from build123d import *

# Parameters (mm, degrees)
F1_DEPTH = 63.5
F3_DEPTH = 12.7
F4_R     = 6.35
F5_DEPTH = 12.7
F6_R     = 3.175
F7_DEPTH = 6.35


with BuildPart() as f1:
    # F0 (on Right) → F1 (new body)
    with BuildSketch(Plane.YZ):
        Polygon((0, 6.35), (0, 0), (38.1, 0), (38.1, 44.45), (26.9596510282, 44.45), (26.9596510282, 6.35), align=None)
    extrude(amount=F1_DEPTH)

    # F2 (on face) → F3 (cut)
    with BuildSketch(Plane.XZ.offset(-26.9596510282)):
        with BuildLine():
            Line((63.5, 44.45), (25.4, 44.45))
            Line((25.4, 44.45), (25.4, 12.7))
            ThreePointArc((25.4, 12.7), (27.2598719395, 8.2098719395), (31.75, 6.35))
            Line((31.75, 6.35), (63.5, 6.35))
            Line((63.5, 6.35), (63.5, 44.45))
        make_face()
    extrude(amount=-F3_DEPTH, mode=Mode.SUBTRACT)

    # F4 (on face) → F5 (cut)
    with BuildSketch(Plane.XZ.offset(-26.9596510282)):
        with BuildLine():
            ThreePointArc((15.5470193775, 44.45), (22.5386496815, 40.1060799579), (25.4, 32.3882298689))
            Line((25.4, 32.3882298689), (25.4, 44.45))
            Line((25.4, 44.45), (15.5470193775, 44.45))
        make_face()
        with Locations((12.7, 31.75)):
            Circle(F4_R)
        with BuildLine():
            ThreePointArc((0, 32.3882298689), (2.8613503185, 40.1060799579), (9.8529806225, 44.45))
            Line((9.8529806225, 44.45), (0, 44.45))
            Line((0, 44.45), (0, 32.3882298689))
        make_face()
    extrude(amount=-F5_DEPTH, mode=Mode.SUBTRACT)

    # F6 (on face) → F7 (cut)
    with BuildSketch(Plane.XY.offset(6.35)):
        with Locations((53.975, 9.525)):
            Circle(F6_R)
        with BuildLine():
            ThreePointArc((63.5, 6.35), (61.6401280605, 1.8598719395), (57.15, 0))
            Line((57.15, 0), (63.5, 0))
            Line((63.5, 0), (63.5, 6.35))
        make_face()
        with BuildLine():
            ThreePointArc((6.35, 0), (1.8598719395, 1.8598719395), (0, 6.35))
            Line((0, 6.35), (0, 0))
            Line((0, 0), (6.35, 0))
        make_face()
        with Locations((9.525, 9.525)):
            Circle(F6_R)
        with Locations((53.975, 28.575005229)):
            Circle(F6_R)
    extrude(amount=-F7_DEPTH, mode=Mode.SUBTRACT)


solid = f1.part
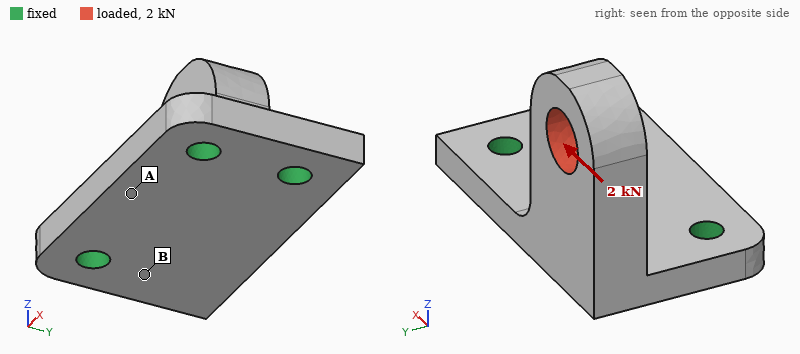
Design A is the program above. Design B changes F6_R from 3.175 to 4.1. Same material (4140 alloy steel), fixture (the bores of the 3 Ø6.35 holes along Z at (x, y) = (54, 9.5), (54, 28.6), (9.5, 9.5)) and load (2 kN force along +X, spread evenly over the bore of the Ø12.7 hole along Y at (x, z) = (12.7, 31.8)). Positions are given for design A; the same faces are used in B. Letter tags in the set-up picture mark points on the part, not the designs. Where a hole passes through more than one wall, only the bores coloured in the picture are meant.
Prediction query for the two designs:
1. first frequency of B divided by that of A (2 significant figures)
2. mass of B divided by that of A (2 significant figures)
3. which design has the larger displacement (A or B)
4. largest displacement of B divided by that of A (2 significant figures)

1.0
0.98
A
0.92
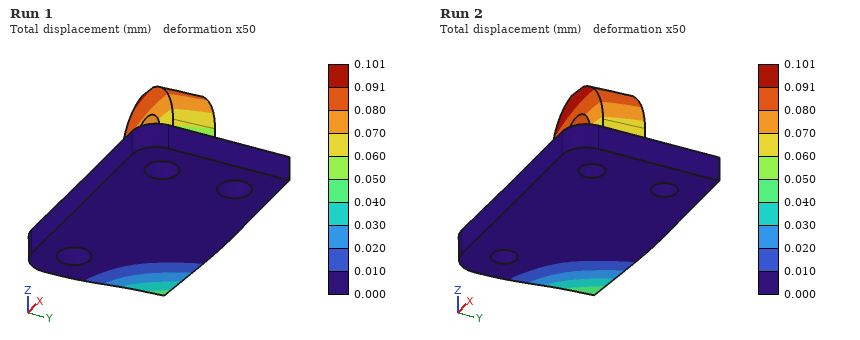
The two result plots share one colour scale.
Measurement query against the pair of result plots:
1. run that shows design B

Run 1
